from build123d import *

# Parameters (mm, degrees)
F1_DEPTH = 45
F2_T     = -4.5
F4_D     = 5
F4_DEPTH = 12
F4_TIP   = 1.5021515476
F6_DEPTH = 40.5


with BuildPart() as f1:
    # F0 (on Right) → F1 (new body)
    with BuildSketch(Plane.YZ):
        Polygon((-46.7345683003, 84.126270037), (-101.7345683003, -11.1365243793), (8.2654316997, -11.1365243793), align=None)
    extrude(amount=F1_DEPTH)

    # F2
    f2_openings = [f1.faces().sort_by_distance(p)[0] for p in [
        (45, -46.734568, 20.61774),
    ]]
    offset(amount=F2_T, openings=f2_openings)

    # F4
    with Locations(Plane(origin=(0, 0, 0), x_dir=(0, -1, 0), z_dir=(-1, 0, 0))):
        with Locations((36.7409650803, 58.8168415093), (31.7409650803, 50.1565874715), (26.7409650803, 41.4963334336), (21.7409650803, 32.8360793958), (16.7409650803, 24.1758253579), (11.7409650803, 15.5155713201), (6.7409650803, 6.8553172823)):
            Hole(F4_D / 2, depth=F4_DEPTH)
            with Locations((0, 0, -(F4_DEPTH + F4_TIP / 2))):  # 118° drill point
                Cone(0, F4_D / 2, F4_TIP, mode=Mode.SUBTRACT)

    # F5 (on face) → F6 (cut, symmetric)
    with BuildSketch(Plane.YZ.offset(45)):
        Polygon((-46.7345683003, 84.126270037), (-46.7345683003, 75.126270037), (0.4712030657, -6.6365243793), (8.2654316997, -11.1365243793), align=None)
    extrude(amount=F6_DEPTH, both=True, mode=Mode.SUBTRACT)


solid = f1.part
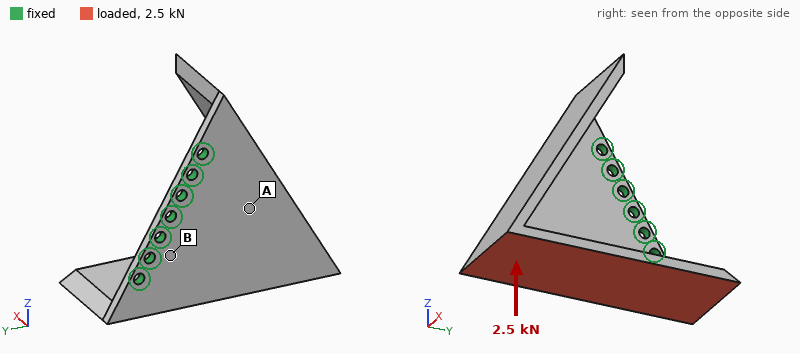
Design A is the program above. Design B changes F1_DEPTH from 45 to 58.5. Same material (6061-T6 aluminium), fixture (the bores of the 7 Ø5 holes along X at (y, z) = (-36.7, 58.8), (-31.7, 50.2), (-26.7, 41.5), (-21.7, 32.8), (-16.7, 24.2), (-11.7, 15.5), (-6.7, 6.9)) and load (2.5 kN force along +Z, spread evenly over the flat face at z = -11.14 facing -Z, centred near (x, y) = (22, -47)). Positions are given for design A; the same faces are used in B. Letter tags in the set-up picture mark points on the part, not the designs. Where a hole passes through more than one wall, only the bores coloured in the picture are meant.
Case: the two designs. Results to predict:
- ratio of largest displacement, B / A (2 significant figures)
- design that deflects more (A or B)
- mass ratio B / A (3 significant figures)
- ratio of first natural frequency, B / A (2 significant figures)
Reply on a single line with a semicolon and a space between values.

1.7; B; 1.21; 0.83
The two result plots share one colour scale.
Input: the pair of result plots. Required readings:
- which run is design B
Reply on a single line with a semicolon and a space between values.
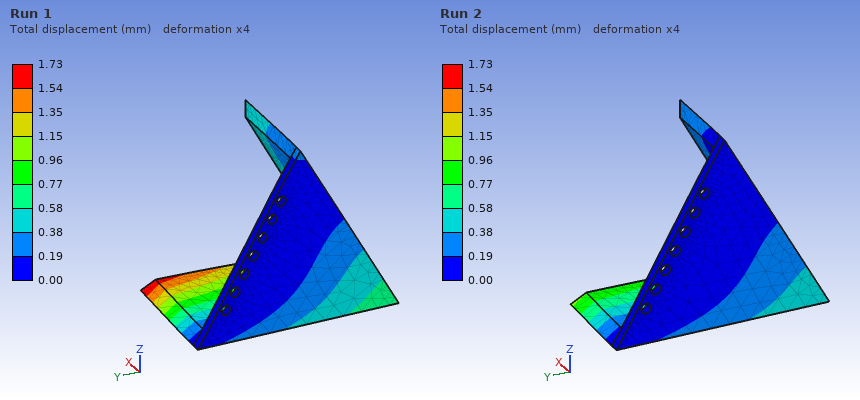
Run 1
